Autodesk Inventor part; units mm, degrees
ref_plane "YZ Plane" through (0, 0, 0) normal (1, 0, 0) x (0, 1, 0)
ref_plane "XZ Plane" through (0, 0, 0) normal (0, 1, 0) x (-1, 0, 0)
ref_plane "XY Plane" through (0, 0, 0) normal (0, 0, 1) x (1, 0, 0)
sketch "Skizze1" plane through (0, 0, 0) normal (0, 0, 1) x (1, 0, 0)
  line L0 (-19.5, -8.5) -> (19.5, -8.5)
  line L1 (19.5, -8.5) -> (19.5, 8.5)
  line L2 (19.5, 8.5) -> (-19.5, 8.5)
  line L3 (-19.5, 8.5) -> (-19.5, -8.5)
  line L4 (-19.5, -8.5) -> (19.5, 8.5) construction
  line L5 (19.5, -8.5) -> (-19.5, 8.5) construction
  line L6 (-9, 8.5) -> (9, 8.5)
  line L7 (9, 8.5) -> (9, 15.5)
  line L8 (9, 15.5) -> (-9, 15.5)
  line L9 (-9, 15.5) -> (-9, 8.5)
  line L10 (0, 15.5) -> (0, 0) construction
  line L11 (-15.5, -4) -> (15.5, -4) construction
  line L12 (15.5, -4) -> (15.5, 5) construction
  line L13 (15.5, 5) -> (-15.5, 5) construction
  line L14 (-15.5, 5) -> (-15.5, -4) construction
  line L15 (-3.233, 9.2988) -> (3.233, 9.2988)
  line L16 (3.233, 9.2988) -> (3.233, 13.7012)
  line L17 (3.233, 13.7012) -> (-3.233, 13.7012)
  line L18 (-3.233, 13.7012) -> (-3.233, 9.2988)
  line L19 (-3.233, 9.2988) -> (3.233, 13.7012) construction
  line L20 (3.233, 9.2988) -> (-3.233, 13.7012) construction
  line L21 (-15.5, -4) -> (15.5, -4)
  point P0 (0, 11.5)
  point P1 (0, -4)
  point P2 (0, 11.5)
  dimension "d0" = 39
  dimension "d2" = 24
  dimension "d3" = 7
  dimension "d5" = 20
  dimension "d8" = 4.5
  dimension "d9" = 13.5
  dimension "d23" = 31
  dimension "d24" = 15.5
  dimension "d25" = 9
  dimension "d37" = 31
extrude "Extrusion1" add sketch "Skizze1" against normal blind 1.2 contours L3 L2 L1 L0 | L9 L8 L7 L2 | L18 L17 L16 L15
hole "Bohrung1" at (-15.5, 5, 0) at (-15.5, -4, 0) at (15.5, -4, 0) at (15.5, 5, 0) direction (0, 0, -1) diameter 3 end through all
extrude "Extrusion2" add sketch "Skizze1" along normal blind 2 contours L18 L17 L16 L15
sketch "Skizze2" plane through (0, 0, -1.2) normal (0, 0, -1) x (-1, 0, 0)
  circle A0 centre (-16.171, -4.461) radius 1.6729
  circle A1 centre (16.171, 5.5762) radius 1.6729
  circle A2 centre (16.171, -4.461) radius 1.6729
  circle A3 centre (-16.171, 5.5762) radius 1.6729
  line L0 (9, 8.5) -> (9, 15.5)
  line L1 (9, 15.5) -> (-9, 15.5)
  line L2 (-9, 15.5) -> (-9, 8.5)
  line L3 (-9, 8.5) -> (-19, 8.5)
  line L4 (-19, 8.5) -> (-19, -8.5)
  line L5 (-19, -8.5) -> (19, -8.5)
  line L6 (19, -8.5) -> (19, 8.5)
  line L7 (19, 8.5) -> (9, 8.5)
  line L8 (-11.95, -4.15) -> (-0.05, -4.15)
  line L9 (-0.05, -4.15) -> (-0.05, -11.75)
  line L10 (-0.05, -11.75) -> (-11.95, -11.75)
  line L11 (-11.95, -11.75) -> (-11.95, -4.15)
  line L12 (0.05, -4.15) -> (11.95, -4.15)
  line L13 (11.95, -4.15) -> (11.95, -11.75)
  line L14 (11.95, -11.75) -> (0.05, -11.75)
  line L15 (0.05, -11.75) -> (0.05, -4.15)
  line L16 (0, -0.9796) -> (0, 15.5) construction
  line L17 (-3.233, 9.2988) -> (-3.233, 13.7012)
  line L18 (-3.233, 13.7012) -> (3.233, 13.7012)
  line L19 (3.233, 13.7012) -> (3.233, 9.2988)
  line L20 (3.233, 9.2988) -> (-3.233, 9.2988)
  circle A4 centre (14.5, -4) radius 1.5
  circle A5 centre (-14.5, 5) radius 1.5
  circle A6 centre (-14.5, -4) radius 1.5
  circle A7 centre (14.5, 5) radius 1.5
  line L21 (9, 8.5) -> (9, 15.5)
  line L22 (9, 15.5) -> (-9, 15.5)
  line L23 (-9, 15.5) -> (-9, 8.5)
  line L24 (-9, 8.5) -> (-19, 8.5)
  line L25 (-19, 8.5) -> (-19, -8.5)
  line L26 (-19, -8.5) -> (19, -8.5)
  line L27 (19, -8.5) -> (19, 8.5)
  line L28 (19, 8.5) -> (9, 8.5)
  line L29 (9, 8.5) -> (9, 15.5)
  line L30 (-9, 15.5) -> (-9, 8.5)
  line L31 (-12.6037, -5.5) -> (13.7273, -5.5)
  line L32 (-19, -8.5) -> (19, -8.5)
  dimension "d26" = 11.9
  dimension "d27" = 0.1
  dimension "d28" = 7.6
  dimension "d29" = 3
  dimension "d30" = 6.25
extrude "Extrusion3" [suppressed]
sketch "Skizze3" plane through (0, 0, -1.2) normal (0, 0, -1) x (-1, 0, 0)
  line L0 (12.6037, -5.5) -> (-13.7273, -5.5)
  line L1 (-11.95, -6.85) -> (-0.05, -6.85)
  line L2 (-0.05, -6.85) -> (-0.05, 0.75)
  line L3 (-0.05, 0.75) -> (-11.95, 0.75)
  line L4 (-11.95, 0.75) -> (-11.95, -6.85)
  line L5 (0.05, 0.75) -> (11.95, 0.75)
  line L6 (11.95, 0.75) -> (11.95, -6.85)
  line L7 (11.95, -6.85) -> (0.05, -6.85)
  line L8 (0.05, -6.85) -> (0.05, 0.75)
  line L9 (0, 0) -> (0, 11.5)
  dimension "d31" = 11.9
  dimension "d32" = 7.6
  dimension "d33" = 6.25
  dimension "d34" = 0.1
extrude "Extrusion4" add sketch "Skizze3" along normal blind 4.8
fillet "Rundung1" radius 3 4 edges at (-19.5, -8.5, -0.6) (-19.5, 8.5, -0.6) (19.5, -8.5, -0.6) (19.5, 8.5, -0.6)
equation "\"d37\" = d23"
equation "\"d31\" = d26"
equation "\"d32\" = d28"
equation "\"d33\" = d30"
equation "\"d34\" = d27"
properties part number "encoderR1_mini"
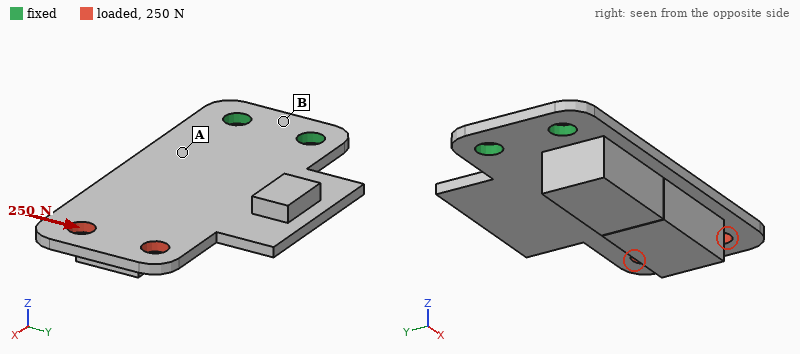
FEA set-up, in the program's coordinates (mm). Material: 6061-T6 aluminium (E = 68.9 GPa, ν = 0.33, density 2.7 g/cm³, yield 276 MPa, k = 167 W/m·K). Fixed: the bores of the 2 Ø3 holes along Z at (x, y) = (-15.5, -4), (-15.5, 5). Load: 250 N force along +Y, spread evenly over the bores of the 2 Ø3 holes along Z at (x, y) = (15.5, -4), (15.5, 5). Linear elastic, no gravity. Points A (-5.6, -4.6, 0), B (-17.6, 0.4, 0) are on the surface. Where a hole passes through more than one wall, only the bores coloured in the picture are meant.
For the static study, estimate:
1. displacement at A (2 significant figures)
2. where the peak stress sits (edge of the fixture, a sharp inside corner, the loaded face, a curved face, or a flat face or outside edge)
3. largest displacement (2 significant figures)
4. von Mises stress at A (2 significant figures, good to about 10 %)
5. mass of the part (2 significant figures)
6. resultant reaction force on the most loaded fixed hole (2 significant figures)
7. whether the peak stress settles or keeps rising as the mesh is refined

0.019 mm
edge of the fixture
0.11 mm
37 MPa
4.9 g
720 N
keeps rising
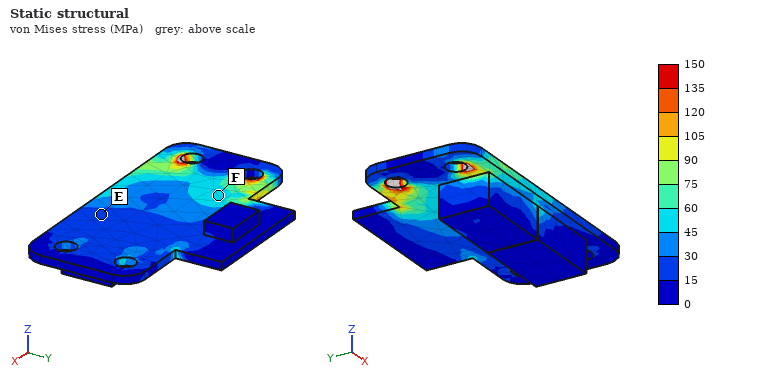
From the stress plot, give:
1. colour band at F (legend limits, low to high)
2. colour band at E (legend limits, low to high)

45 to 60 MPa
15 to 30 MPa
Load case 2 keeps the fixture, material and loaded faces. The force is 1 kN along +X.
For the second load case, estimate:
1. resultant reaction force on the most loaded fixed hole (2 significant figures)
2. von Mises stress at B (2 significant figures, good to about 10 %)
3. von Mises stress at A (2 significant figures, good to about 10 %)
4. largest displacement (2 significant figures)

500 N
9.2 MPa
37 MPa
86 µm
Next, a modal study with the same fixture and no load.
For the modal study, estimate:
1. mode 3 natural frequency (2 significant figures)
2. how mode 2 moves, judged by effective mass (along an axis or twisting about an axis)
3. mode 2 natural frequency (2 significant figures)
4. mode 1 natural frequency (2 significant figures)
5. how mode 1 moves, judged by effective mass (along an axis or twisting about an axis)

6900 Hz
twisting about X
4000 Hz
960 Hz
along Z
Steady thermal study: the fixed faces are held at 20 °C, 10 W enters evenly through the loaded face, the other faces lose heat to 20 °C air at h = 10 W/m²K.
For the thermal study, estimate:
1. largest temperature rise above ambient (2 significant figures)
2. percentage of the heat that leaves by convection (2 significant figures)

61 K
5.4 %
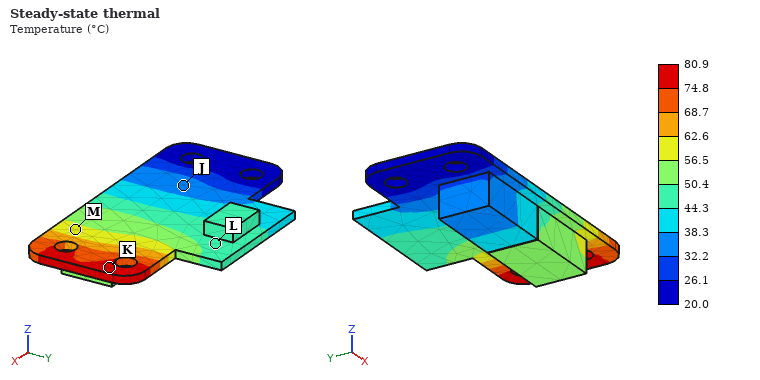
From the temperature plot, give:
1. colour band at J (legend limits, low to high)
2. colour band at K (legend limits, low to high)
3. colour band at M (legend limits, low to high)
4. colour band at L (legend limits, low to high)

32.2 to 38.3 °C
74.8 to 80.9 °C
56.5 to 62.6 °C
44.3 to 50.4 °C
